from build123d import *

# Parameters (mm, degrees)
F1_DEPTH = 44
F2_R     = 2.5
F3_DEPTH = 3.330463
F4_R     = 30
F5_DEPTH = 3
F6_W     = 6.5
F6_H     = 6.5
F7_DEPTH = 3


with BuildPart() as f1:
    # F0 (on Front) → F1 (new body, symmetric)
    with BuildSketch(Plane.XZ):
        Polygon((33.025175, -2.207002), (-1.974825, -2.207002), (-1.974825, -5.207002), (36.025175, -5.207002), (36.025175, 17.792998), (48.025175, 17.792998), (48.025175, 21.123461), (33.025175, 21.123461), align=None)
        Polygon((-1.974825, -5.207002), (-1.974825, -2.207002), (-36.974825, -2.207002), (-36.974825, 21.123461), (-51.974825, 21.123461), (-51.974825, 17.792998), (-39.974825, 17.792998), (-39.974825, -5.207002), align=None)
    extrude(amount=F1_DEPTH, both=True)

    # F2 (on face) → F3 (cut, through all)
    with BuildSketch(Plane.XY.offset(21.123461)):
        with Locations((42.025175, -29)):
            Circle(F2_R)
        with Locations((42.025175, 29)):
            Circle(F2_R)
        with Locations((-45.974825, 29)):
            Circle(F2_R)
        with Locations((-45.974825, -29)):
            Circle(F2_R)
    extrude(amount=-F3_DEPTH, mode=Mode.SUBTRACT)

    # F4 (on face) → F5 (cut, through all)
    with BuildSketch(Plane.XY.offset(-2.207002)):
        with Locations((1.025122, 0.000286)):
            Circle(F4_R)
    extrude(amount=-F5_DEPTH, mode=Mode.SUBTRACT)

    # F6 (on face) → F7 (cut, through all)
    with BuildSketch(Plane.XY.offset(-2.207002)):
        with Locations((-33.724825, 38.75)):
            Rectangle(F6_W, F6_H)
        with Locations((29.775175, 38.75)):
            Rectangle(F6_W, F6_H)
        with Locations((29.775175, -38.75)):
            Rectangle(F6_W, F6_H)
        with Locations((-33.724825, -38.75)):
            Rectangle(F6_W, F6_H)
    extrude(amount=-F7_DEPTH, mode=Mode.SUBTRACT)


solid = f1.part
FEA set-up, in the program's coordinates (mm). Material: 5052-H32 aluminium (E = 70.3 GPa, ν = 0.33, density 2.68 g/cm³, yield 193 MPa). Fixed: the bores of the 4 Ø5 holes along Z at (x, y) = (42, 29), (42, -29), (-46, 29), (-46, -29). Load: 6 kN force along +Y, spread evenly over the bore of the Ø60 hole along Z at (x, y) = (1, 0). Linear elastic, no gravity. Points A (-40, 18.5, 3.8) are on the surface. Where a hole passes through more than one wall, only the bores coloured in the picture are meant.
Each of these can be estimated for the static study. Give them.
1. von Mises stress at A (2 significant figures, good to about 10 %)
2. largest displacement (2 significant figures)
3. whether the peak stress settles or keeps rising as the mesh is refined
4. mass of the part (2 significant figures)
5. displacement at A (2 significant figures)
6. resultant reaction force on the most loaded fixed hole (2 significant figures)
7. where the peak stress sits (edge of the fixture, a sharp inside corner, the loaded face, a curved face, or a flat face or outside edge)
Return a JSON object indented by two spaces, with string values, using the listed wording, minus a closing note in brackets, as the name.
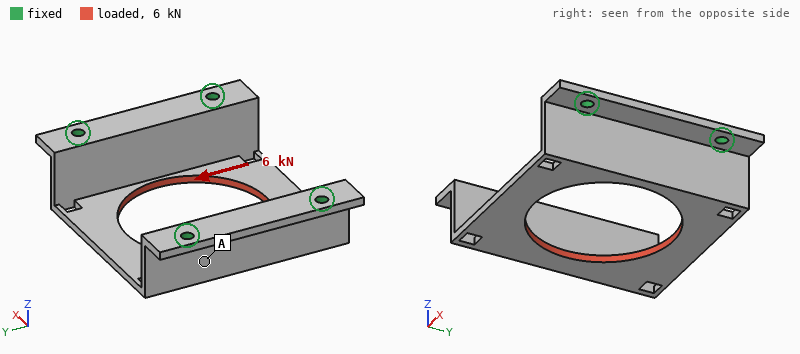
{
  "von Mises stress at A": "15 MPa",
  "largest displacement": "95 µm",
  "whether the peak stress settles or keeps rising as the mesh is refined": "keeps rising",
  "mass of the part": "81 g",
  "displacement at A": "27 µm",
  "resultant reaction force on the most loaded fixed hole": "2.0 kN",
  "where the peak stress sits": "edge of the fixture"
}
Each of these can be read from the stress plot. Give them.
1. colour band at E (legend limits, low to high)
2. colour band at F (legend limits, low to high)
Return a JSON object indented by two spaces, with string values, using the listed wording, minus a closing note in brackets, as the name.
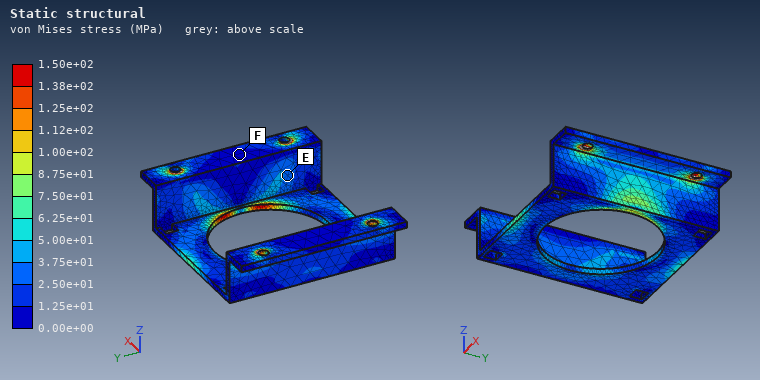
{
  "colour band at E": "2.50e+01 to 3.75e+01 MPa",
  "colour band at F": "0.00e+00 to 1.25e+01 MPa"
}
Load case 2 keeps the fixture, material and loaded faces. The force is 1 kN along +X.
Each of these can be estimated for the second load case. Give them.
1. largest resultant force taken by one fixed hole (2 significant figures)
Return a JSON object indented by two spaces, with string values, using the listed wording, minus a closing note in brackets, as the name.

{
  "largest resultant force taken by one fixed hole": "260 N"
}
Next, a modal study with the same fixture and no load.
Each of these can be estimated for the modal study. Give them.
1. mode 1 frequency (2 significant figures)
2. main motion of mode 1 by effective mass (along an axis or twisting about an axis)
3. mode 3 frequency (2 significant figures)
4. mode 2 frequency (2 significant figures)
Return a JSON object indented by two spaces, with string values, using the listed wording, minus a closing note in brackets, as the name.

{
  "mode 1 frequency": "2000 Hz",
  "main motion of mode 1 by effective mass": "along X",
  "mode 3 frequency": "2700 Hz",
  "mode 2 frequency": "2700 Hz"
}
